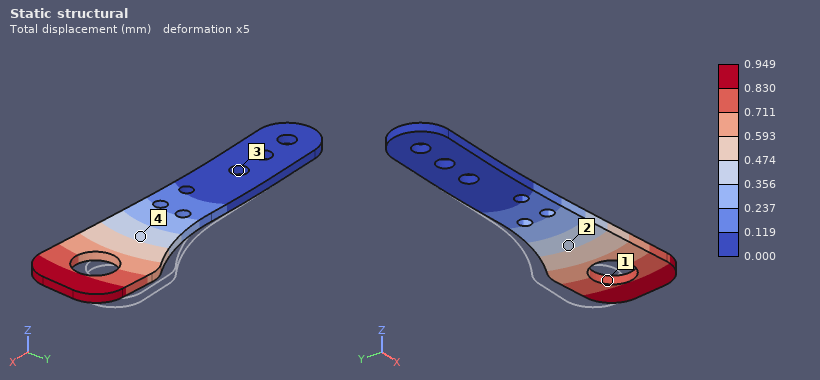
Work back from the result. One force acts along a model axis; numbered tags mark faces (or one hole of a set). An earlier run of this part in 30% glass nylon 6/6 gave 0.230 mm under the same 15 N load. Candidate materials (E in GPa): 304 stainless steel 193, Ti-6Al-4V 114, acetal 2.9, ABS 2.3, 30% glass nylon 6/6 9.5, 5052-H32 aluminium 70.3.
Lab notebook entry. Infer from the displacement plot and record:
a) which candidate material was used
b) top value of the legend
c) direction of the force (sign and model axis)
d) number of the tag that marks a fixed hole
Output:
ABS
0.949 mm
-Y
3
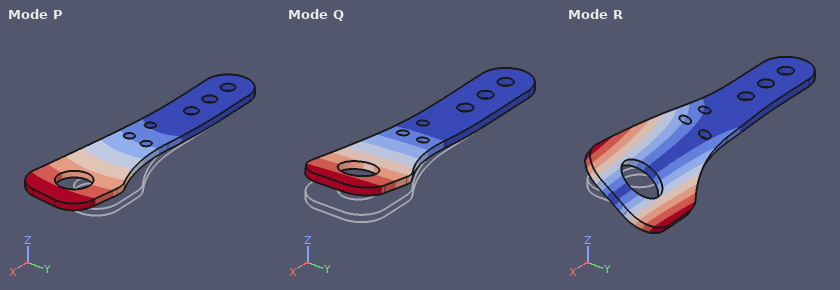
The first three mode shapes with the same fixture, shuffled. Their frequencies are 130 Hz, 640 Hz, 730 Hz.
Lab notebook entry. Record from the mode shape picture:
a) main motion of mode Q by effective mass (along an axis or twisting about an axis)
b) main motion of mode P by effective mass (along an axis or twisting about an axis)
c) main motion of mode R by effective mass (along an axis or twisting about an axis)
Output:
along Z
along Y
twisting about X
